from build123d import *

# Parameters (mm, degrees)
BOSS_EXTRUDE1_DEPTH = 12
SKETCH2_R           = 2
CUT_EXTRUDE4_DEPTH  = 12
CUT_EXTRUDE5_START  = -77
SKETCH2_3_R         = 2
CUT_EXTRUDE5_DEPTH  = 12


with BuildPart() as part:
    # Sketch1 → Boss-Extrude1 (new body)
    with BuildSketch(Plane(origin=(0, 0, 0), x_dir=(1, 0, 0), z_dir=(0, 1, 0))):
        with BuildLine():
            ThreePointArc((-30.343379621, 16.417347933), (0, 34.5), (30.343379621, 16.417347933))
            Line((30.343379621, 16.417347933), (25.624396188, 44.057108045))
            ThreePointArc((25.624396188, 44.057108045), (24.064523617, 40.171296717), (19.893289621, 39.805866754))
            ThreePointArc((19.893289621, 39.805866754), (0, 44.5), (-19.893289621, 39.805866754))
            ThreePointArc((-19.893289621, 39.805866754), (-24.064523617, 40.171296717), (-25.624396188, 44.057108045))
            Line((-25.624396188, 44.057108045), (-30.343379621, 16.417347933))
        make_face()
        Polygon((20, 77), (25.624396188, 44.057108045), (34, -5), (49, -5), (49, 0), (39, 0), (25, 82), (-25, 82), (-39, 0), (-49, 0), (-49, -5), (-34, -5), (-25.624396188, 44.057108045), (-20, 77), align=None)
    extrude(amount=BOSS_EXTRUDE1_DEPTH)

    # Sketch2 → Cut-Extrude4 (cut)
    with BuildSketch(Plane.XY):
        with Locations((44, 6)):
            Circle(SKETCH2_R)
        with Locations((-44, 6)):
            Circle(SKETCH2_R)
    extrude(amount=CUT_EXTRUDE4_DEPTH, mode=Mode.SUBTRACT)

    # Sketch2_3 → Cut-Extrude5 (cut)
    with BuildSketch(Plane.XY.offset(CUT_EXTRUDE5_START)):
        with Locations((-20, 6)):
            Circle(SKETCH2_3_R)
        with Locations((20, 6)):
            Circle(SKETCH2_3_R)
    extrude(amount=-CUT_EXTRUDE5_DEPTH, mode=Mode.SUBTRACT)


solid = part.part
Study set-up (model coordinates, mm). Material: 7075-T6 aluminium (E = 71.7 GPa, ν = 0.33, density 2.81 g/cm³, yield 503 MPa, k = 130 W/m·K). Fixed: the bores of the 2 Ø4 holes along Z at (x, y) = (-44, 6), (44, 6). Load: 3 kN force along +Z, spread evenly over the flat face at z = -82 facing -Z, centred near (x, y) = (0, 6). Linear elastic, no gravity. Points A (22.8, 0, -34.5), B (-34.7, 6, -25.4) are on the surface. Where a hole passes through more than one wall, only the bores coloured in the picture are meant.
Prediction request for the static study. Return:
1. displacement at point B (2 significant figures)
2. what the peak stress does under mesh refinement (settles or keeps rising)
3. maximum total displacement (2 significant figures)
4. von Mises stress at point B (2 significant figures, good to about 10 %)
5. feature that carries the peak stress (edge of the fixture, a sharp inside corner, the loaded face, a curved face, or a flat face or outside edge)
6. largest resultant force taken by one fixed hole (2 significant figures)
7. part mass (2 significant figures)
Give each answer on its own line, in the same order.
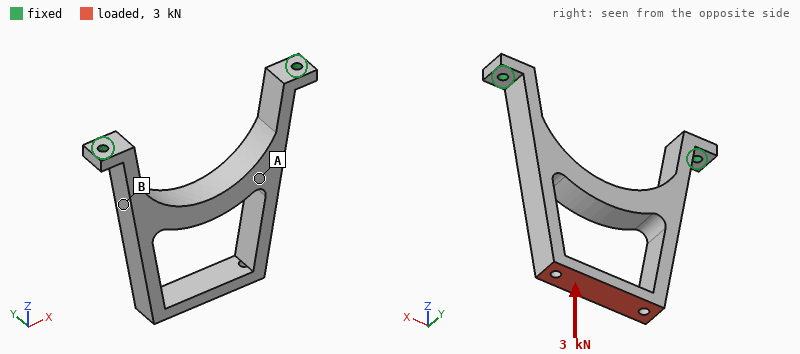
0.031 mm
keeps rising
0.20 mm
31 MPa
a sharp inside corner
1.5 kN
66 g
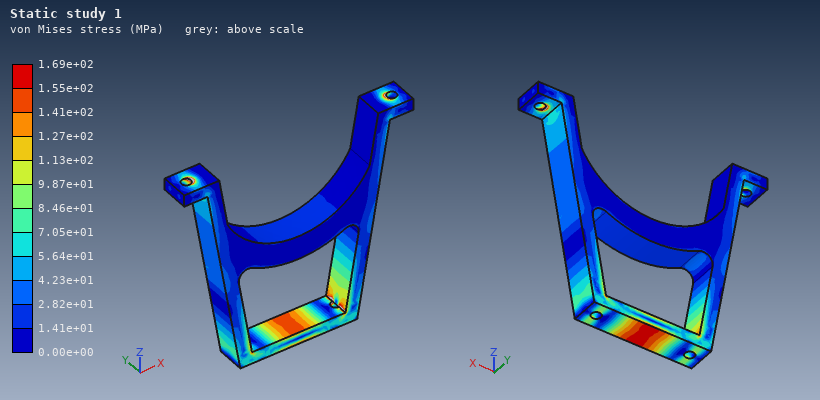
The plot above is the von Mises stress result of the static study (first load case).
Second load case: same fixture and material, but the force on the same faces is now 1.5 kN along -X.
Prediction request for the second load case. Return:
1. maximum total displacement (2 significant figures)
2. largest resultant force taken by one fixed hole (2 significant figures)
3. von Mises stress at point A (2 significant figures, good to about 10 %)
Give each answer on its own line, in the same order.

0.59 mm
1.7 kN
33 MPa
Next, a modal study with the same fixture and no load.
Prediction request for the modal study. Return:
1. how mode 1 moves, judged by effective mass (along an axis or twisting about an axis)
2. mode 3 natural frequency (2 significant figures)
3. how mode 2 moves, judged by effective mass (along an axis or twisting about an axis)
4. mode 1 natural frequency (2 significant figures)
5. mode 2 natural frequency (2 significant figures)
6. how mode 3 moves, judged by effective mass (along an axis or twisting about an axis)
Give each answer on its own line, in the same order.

along Y
2100 Hz
along X
640 Hz
2000 Hz
twisting about Z
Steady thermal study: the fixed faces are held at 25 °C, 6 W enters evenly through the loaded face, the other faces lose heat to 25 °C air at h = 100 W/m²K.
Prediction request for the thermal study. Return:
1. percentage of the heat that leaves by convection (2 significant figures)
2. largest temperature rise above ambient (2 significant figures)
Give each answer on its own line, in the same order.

78 %
14 K
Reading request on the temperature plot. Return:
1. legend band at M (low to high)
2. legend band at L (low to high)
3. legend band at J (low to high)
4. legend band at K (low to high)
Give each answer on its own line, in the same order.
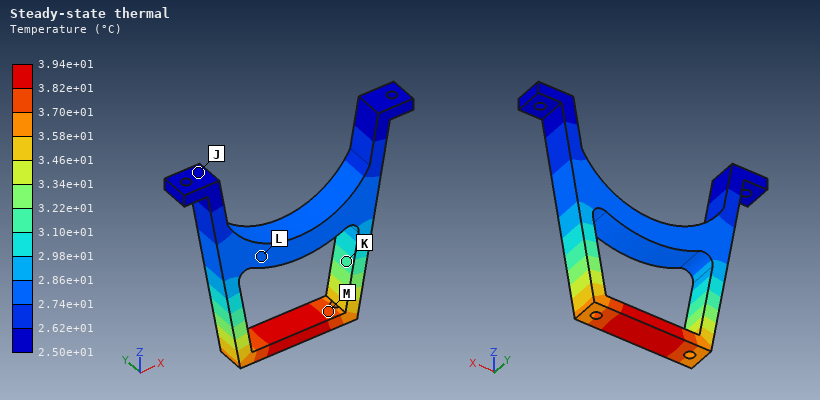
3.70e+01 to 3.82e+01 °C
2.74e+01 to 2.86e+01 °C
2.50e+01 to 2.62e+01 °C
3.10e+01 to 3.22e+01 °C
